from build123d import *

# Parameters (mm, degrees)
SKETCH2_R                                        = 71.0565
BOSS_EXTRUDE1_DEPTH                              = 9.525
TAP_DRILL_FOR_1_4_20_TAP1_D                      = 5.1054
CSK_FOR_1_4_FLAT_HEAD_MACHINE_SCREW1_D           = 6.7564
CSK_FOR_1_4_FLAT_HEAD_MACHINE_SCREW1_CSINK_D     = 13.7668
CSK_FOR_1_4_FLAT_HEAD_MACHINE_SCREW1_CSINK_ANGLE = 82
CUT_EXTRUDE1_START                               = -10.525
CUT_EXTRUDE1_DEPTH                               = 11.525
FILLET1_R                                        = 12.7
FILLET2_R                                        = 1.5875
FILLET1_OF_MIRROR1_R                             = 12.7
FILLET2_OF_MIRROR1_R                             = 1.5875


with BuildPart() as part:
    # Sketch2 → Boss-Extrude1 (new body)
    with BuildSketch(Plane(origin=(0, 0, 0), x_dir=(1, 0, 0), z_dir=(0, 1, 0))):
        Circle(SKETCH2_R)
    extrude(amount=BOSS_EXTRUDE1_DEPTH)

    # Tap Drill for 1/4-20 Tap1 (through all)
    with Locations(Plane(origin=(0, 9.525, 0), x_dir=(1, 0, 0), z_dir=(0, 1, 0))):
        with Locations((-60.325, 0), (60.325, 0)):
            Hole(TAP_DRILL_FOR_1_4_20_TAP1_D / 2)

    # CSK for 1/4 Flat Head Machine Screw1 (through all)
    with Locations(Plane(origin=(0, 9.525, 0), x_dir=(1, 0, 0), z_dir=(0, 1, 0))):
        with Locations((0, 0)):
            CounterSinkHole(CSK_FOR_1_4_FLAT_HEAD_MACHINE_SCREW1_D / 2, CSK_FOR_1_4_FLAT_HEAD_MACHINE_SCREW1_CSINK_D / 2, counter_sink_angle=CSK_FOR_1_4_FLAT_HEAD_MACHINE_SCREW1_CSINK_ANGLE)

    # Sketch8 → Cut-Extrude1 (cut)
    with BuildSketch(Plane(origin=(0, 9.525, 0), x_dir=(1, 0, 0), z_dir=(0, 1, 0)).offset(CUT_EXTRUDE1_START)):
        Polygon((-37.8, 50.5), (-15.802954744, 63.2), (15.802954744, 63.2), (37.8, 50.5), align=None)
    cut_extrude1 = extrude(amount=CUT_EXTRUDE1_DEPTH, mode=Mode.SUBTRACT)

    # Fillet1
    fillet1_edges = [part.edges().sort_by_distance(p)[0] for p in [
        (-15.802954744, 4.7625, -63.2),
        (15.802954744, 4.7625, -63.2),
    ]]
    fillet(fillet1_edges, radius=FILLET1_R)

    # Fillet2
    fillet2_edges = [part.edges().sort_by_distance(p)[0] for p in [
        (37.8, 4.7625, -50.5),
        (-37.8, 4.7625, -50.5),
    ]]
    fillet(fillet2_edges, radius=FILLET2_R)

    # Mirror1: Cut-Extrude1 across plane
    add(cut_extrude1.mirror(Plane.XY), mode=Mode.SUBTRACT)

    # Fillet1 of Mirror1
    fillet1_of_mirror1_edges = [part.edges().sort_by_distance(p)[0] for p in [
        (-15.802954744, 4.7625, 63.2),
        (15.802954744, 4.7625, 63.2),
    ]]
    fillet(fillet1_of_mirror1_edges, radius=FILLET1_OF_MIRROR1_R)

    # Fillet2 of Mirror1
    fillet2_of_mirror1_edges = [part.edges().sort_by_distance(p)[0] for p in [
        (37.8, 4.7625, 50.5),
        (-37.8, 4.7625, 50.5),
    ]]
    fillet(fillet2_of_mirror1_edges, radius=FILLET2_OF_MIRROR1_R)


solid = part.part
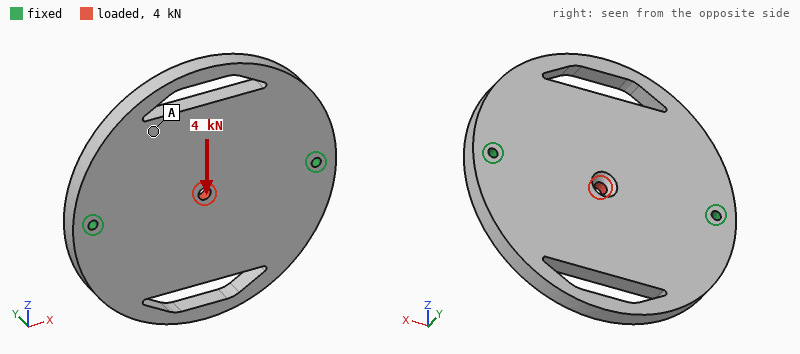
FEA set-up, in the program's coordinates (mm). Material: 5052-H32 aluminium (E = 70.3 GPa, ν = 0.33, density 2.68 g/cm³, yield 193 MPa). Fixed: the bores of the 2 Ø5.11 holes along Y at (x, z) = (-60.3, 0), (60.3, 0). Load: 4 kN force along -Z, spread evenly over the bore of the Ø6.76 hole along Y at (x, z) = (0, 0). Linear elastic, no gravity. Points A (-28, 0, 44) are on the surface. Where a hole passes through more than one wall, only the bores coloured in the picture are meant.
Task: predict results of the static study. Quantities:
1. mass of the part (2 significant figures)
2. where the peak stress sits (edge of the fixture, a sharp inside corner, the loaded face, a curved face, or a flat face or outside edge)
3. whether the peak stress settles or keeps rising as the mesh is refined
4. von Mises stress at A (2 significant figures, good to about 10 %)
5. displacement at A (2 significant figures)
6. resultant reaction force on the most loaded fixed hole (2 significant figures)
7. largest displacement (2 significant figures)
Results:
370 g
edge of the fixture
keeps rising
3.8 MPa
17 µm
2.0 kN
26 µm
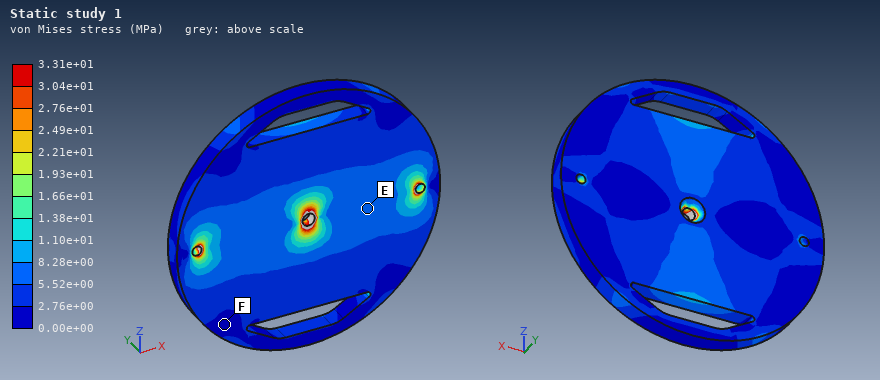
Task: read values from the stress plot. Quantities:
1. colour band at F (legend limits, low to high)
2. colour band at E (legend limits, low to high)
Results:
0.00e+00 to 2.76e+00 MPa
5.52e+00 to 8.28e+00 MPa
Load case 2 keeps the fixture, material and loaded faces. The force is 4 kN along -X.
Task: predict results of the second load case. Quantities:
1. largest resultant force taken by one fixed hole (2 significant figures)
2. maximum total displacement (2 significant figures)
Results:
2.0 kN
9.1 µm
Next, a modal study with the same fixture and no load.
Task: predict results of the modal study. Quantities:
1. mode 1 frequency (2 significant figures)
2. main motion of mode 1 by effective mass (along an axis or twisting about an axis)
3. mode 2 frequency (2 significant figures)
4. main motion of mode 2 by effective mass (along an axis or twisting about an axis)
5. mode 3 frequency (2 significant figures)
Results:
1200 Hz
twisting about X
1700 Hz
along Y
3400 Hz
